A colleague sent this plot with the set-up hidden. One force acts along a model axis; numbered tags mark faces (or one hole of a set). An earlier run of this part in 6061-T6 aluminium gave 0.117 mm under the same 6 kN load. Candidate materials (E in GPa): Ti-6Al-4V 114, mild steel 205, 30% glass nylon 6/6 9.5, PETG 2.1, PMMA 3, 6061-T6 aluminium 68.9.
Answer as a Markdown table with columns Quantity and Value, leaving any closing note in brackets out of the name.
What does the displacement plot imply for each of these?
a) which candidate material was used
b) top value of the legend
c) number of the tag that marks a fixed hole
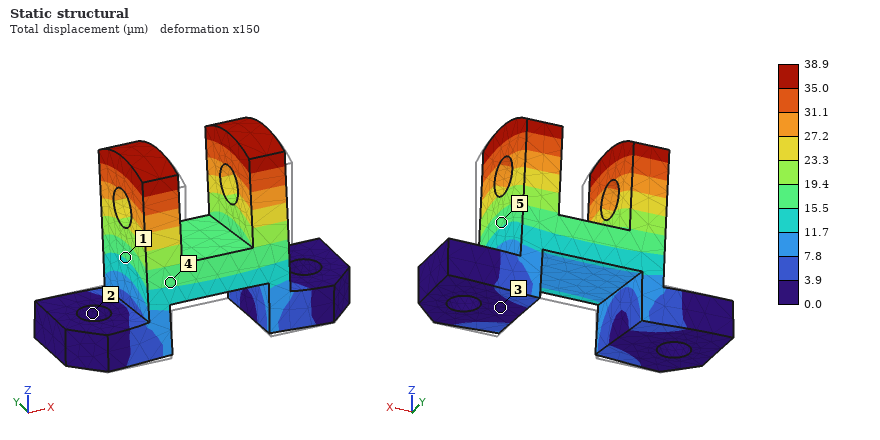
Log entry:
| Quantity | Value |
|---|---|
| which candidate material was used | mild steel |
| top value of the legend | 38.9 µm |
| number of the tag that marks a fixed hole | 2 |
